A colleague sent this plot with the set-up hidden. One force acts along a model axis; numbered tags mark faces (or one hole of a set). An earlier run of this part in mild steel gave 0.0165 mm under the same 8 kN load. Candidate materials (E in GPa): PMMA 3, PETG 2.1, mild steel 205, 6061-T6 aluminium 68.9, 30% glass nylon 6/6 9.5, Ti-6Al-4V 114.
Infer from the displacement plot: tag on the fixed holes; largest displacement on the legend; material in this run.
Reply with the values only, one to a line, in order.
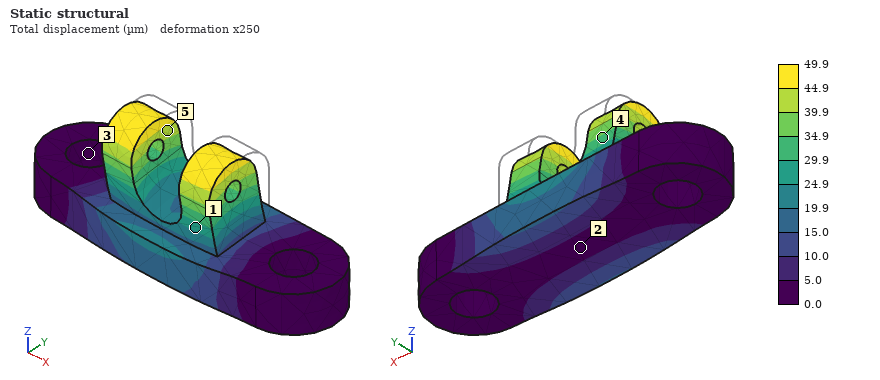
3
49.9 µm
6061-T6 aluminium
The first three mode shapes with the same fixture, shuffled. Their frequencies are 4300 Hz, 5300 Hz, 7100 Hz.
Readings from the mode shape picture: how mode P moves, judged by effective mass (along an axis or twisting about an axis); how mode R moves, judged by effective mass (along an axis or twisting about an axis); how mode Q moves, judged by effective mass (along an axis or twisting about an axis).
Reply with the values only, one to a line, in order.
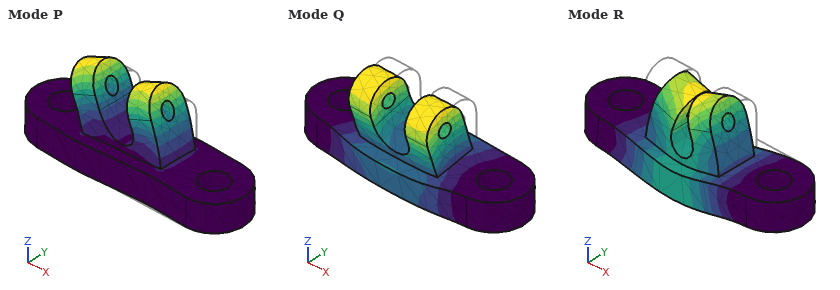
along X
along Z
along Y
